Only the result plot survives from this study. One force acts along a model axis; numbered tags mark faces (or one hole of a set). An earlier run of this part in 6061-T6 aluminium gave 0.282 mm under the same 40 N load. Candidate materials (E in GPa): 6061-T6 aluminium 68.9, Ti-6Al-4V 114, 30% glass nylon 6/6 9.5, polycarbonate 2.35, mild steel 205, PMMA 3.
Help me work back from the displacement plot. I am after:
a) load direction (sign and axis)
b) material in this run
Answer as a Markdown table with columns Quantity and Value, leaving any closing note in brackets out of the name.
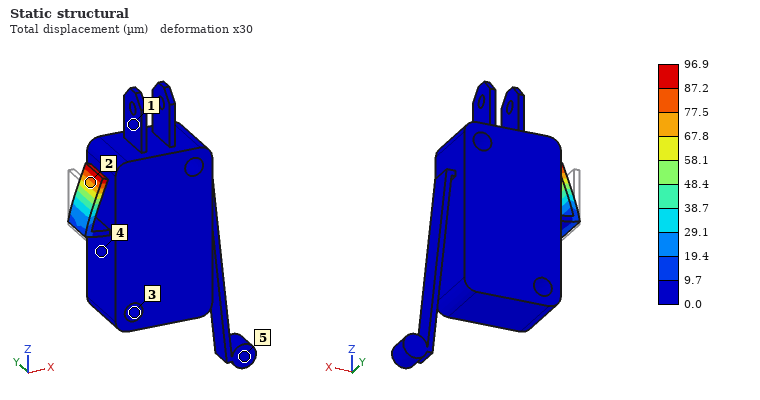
| Quantity | Value |
|---|---|
| load direction | +X |
| material in this run | mild steel |
